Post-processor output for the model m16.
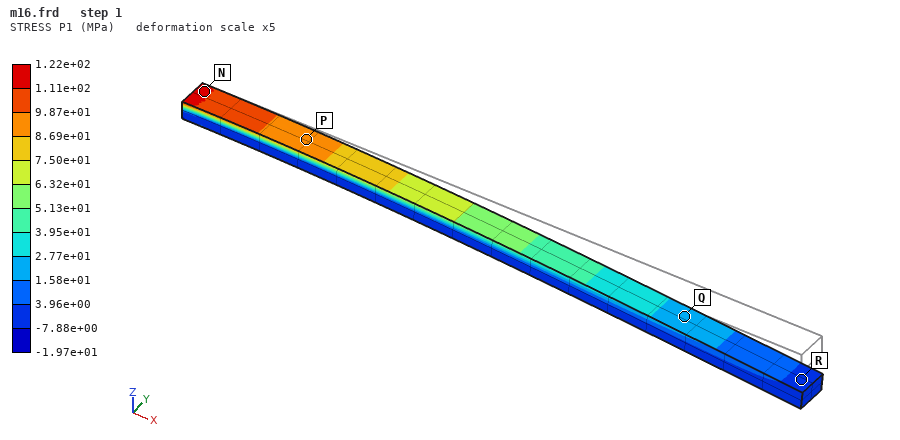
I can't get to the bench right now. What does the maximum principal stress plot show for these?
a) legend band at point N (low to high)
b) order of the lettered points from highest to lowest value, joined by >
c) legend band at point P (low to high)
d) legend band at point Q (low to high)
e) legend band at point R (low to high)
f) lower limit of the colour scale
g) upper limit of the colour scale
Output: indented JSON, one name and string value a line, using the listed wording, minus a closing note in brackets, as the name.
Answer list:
{
  "legend band at point N": "1.11e+02 to 1.22e+02 MPa",
  "order of the lettered points from highest to lowest value, joined by >": "N > P > Q > R",
  "legend band at point P": "8.69e+01 to 9.87e+01 MPa",
  "legend band at point Q": "1.58e+01 to 2.77e+01 MPa",
  "legend band at point R": "-7.88e+00 to 3.96e+00 MPa",
  "lower limit of the colour scale": "-1.97e+01 MPa",
  "upper limit of the colour scale": "1.22e+02 MPa"
}
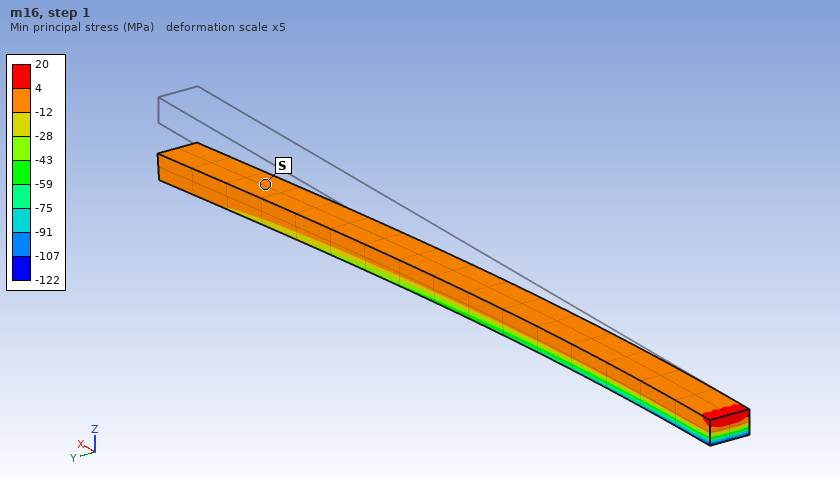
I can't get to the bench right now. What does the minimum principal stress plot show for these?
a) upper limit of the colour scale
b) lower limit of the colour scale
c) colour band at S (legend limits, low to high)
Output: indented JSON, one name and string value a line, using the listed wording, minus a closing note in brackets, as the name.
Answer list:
{
  "upper limit of the colour scale": "20 MPa",
  "lower limit of the colour scale": "-122 MPa",
  "colour band at S": "-12 to 4 MPa"
}
